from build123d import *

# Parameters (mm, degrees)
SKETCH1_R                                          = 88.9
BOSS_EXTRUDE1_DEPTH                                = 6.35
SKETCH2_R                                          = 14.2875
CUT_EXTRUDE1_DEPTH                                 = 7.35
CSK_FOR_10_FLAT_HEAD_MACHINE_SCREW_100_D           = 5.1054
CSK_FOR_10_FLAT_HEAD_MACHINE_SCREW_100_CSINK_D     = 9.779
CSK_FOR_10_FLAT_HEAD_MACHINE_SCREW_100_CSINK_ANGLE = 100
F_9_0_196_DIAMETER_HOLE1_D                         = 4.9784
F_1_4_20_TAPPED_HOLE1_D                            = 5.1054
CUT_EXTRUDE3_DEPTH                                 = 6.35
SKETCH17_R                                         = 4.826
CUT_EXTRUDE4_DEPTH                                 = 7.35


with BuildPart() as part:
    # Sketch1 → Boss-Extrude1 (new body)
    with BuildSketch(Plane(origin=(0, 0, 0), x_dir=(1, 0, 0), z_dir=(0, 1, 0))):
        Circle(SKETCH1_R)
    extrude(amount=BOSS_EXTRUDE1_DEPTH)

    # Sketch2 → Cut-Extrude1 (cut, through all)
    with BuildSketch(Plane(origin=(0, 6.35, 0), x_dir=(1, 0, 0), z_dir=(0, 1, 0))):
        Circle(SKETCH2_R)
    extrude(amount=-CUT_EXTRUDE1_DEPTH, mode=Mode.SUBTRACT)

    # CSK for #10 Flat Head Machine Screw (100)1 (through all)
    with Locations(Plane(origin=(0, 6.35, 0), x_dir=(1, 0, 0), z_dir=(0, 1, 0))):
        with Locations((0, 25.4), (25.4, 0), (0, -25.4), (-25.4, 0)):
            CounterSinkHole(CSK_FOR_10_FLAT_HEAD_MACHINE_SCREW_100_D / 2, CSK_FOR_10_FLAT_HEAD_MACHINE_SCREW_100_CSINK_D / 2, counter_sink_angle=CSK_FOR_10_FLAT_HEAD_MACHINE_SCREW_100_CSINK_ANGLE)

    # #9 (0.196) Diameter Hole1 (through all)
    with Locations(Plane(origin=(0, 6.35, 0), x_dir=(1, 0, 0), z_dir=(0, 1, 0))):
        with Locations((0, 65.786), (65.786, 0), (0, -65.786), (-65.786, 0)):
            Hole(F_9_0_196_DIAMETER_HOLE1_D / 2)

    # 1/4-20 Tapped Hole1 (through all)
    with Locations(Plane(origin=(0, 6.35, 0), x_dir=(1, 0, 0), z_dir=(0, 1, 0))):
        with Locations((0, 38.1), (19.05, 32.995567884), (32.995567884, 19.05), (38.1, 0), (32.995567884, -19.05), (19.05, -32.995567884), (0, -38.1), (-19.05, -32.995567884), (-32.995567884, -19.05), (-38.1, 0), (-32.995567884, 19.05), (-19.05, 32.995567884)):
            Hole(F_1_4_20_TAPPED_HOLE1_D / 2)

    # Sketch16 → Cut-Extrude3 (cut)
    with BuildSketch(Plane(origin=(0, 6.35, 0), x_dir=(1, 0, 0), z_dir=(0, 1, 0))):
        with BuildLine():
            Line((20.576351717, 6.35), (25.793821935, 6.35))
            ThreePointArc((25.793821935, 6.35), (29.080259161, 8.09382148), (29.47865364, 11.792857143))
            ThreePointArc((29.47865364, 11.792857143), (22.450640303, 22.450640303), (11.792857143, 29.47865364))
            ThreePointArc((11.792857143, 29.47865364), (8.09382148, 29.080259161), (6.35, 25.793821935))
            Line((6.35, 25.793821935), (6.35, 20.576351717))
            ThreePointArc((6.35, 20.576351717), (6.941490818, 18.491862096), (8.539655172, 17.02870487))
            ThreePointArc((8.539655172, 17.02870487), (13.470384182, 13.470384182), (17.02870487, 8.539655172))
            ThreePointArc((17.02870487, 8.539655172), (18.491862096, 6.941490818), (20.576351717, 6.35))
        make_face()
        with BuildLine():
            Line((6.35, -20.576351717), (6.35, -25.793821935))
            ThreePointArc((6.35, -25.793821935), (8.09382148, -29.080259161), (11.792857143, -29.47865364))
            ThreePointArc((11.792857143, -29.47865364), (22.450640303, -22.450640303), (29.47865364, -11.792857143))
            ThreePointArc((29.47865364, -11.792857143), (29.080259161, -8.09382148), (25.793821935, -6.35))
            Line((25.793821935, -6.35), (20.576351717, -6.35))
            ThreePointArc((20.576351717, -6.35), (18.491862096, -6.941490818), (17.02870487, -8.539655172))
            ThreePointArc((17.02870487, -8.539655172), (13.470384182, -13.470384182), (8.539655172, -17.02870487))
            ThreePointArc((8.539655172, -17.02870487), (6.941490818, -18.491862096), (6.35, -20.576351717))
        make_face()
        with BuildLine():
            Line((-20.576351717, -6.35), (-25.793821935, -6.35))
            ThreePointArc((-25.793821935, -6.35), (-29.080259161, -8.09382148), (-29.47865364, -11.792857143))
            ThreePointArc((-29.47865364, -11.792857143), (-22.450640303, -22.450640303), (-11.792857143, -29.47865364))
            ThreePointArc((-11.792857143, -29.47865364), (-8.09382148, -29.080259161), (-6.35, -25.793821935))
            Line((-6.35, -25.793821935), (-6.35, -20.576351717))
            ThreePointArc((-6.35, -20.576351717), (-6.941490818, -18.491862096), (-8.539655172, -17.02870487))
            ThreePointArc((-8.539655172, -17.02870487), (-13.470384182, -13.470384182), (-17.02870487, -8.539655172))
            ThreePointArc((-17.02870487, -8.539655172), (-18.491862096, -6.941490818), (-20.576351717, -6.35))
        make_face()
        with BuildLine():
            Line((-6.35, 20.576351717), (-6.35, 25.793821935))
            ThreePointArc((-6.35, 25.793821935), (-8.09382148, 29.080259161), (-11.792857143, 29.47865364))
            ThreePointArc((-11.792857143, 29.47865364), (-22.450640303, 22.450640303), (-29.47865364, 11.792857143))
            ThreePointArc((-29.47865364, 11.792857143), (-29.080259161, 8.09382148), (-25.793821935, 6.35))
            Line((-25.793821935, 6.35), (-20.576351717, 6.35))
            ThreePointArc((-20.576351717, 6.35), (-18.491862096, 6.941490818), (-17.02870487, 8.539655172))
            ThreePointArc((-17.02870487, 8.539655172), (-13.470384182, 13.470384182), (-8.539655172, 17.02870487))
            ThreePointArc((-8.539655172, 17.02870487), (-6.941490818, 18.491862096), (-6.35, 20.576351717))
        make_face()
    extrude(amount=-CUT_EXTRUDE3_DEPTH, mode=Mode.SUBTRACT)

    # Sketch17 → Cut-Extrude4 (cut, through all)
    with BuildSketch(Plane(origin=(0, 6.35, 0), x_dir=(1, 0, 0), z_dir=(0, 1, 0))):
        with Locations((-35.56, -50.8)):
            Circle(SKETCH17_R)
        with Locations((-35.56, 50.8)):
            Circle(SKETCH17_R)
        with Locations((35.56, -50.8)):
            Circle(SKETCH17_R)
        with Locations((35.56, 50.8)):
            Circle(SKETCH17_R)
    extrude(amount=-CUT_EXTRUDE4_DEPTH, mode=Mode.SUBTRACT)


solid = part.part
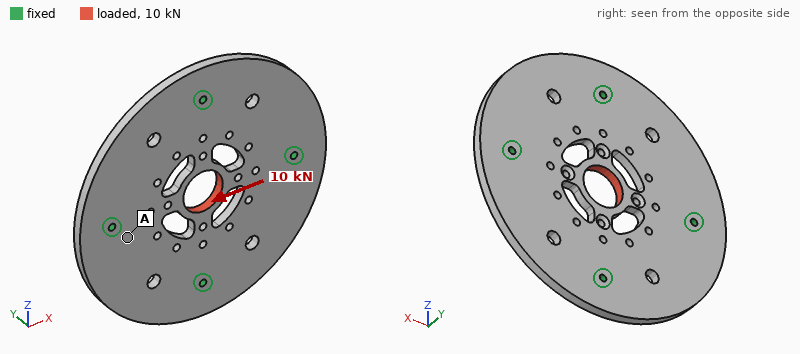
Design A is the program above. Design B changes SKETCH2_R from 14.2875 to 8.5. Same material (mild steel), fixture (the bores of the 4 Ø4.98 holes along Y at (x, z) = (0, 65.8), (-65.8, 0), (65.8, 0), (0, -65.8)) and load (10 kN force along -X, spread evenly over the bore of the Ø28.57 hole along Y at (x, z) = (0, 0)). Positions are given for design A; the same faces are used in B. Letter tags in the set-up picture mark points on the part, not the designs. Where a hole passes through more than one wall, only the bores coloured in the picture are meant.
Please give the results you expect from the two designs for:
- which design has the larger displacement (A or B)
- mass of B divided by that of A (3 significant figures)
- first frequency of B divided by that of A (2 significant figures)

A
1.02
1.0
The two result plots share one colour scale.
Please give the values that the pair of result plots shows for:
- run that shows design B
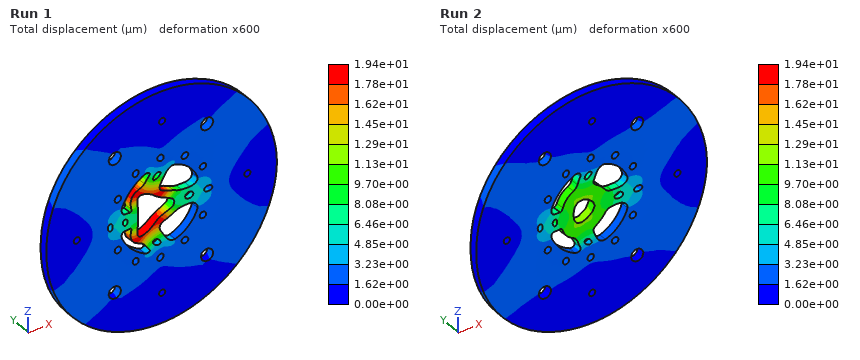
Run 2
